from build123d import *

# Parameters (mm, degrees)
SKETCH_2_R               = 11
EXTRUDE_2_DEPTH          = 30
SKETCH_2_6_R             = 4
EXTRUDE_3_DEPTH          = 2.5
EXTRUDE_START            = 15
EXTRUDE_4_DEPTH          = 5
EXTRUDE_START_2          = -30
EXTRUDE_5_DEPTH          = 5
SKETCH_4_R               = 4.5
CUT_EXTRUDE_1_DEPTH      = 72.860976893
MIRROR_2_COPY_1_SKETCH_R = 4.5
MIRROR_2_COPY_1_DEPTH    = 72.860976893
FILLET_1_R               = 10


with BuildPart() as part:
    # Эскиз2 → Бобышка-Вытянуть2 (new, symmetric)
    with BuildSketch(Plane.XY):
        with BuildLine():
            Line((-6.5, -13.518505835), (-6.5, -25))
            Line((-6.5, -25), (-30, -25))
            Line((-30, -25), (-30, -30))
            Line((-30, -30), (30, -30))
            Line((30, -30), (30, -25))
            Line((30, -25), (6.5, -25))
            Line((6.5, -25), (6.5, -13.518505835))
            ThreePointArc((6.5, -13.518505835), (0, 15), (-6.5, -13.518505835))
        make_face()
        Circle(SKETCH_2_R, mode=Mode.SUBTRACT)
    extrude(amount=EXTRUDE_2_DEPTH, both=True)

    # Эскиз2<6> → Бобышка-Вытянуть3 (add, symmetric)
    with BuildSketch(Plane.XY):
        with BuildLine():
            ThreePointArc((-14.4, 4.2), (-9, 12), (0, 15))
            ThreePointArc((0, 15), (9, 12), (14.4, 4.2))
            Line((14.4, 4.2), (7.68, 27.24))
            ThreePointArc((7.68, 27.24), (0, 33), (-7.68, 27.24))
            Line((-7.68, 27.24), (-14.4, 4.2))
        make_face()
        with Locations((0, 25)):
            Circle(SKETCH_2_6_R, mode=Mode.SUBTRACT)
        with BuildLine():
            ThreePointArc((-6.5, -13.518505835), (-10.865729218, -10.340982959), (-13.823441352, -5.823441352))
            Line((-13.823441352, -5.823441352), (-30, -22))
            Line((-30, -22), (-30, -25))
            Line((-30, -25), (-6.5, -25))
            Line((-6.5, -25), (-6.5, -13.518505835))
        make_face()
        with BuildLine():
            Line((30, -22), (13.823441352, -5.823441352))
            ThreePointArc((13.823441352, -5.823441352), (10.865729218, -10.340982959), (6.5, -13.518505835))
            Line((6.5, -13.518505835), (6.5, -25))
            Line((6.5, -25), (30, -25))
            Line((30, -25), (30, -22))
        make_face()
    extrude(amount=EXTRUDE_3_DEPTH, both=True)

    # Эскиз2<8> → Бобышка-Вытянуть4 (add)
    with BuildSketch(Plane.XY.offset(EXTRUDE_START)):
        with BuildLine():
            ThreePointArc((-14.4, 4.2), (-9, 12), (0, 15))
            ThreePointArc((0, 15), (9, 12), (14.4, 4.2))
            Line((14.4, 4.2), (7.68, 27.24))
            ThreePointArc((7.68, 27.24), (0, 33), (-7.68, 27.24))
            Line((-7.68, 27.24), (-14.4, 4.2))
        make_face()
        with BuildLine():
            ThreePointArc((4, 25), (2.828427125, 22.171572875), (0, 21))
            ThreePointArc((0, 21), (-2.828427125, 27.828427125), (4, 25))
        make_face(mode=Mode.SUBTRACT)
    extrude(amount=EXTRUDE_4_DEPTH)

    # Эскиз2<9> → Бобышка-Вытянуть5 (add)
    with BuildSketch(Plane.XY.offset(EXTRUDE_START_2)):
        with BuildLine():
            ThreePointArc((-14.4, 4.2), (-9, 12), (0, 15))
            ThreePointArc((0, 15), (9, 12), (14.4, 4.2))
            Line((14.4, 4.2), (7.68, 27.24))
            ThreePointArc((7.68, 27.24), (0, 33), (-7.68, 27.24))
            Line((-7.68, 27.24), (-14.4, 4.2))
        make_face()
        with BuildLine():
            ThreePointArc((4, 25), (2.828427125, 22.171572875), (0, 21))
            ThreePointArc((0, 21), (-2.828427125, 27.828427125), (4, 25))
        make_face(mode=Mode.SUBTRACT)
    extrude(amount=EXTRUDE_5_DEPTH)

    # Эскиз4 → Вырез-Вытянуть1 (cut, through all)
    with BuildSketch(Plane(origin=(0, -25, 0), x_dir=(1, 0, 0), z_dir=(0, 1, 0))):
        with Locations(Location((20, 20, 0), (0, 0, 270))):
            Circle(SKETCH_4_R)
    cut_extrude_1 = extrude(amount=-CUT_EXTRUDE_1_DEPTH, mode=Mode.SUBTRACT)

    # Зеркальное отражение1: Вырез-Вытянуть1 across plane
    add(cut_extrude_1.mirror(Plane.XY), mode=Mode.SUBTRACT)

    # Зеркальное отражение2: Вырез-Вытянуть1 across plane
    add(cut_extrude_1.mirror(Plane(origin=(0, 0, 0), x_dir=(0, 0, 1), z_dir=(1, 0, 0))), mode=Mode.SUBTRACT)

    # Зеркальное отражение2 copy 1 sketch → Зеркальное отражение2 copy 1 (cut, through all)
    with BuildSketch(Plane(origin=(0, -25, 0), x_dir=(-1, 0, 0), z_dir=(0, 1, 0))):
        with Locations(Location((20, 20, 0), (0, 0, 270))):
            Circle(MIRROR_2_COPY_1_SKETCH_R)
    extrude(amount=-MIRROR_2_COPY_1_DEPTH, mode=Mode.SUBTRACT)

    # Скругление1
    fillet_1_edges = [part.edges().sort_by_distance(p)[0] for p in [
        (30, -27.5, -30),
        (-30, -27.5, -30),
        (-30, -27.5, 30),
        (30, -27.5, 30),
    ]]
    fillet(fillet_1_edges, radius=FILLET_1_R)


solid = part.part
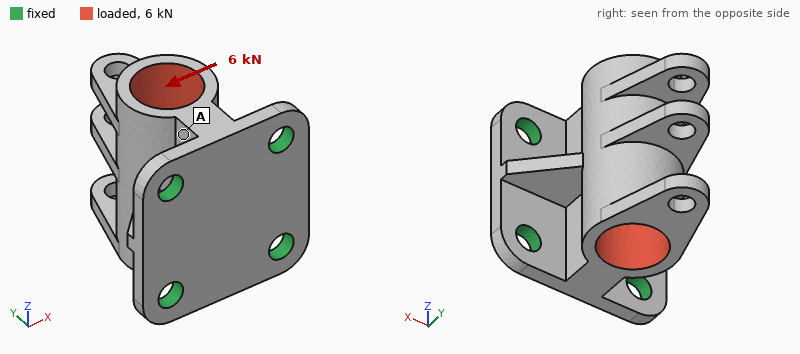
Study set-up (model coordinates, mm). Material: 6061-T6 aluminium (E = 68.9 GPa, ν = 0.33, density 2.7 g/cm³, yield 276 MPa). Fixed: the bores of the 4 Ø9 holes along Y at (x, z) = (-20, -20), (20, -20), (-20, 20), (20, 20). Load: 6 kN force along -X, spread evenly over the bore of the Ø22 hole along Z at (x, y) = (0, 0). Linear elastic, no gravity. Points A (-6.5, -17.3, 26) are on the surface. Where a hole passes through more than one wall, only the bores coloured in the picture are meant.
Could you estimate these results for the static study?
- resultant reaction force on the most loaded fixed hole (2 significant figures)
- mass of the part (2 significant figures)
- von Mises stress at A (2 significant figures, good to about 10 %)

2.8 kN
140 g
23 MPa
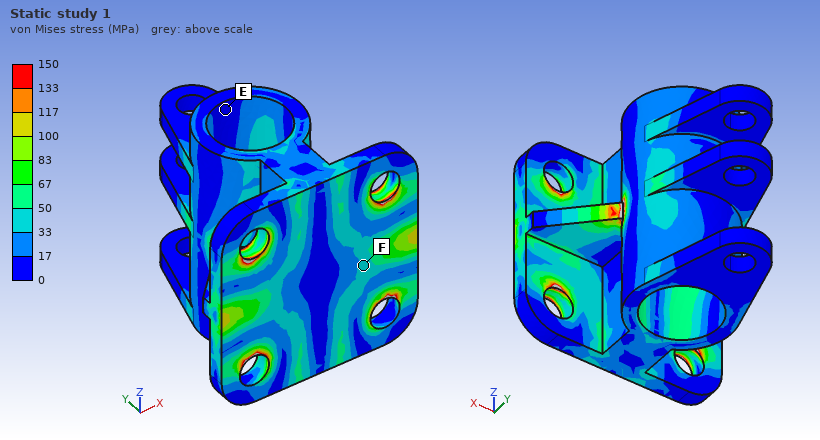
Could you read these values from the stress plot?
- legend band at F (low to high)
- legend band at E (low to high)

33 to 50 MPa
0 to 17 MPa
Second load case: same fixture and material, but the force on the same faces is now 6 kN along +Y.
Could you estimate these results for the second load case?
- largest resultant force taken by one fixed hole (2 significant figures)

1.6 kN
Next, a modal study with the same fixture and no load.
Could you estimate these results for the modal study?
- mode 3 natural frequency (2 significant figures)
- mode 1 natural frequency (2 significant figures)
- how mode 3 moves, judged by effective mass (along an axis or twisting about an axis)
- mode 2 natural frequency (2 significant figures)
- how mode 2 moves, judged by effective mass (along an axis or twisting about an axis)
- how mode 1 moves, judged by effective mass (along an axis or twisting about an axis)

7800 Hz
3500 Hz
along Y
4200 Hz
along Z
along X
